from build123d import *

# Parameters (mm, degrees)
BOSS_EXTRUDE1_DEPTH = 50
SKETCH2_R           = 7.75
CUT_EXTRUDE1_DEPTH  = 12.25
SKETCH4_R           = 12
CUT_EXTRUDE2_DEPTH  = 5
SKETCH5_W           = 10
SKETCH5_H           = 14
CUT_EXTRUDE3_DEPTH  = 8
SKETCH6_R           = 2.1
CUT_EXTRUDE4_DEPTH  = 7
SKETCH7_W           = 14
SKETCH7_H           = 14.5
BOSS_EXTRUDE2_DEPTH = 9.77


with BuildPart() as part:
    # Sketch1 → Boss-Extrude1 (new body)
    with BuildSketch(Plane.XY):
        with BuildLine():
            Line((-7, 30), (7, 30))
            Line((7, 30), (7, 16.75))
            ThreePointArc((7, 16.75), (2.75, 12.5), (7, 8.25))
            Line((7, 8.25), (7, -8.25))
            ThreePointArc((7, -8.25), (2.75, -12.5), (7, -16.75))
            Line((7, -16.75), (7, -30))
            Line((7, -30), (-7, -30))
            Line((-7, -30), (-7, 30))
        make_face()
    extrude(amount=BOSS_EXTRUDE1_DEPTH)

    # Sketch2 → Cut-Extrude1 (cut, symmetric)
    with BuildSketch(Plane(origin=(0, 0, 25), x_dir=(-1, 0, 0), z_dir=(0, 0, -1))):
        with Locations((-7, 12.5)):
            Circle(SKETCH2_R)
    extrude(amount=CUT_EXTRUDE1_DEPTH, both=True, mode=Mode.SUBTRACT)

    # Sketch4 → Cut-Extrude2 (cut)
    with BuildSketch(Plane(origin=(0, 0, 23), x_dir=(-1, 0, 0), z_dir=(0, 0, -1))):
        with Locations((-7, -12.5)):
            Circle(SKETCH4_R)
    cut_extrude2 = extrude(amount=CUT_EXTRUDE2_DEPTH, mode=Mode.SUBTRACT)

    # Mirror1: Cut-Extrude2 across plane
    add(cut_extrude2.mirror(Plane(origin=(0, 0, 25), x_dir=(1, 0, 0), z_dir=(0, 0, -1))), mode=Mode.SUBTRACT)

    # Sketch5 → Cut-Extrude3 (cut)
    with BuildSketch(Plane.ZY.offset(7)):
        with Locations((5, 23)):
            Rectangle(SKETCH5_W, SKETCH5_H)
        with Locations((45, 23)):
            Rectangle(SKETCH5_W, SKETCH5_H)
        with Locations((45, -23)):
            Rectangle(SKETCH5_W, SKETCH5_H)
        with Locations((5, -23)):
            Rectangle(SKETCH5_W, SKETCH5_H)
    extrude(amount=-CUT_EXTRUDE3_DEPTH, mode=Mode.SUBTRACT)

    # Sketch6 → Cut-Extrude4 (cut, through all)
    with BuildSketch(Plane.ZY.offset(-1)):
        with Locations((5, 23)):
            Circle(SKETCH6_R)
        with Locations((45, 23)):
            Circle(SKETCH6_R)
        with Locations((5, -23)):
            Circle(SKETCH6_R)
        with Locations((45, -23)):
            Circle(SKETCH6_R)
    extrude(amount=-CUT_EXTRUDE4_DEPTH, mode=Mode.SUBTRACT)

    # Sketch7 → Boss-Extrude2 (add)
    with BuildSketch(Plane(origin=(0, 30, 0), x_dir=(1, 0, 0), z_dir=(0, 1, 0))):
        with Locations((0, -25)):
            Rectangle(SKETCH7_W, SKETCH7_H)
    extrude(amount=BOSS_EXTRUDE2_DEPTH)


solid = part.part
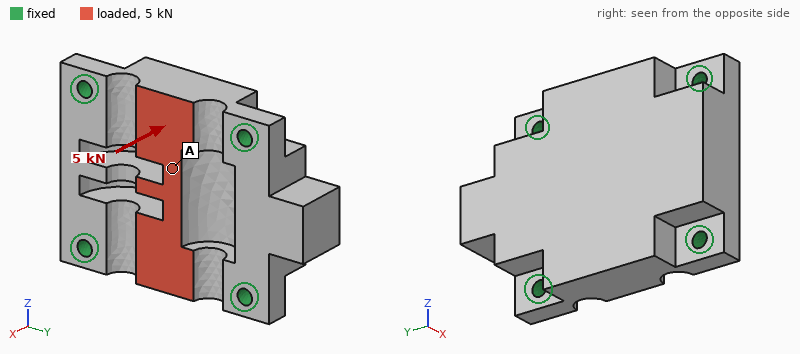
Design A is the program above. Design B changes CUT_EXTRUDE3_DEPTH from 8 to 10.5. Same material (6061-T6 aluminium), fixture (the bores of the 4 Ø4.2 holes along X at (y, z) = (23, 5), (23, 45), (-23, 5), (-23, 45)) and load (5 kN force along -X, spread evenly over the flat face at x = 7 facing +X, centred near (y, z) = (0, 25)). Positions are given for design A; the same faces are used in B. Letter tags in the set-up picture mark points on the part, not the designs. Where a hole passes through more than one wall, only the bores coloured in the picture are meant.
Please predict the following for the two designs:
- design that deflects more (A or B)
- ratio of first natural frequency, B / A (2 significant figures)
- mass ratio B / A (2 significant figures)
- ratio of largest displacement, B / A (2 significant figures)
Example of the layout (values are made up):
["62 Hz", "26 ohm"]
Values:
["B", "0.76", "0.96", "1.6"]
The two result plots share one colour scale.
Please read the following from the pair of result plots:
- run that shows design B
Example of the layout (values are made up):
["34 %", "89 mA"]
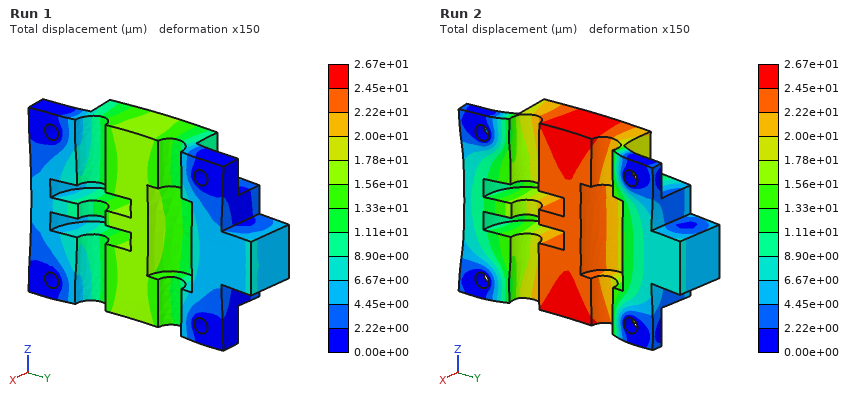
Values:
["Run 2"]
